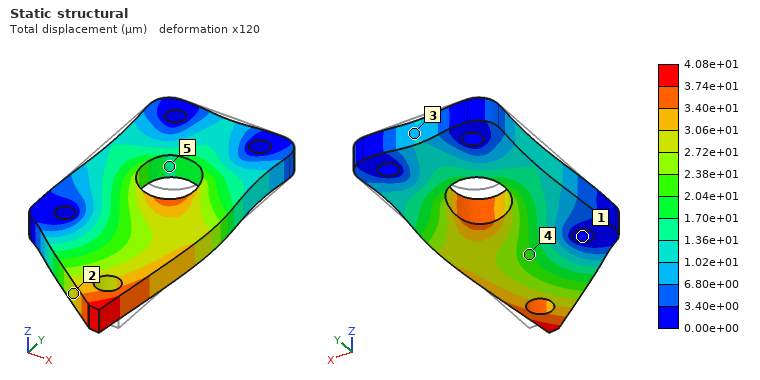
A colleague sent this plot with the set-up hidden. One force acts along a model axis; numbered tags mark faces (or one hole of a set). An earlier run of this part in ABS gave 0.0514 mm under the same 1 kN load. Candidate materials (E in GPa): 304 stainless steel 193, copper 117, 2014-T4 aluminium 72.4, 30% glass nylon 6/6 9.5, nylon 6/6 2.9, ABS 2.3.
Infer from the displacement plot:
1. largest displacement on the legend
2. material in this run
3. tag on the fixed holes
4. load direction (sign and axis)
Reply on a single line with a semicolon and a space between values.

4.08e+01 µm; nylon 6/6; 1; -Y
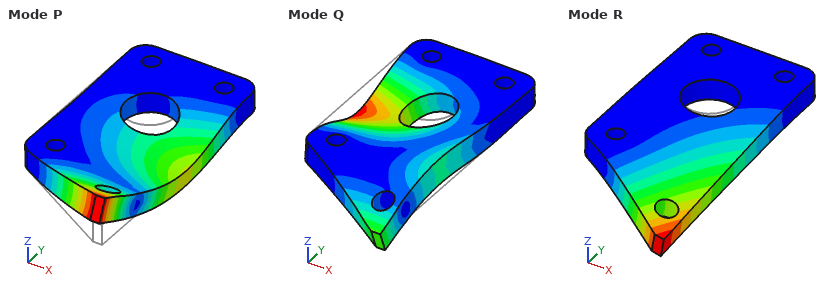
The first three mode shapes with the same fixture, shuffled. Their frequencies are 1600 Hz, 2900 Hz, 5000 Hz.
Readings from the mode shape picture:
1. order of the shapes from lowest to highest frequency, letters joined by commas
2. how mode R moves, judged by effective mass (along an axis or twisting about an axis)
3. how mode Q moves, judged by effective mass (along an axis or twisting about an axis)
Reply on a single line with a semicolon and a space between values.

R, P, Q; along Z; along Z
